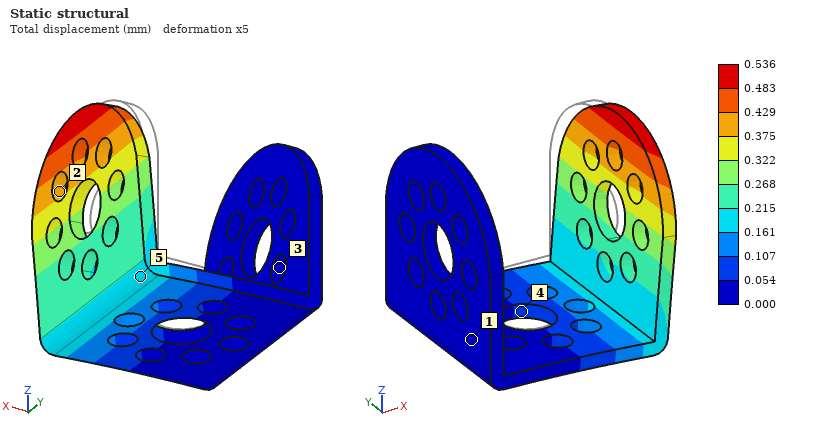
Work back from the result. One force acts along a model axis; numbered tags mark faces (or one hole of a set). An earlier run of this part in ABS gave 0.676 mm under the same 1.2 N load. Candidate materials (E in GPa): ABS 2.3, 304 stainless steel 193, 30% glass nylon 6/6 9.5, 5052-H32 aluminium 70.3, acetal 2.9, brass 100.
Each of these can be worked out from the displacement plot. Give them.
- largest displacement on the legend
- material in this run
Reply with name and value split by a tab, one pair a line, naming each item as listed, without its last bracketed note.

largest displacement on the legend	0.536 mm
material in this run	acetal
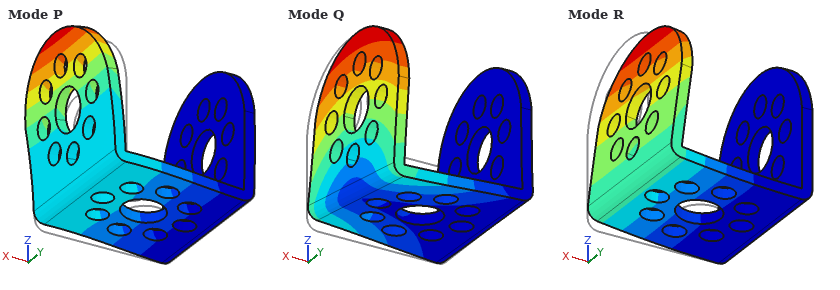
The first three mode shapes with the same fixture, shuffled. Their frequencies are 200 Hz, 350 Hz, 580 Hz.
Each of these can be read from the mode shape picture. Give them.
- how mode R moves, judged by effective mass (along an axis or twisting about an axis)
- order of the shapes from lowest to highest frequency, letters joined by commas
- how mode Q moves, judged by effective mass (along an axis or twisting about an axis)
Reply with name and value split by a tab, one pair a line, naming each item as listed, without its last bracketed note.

how mode R moves, judged by effective mass	along Z
order of the shapes from lowest to highest frequency, letters joined by commas	R, Q, P
how mode Q moves, judged by effective mass	along Y
